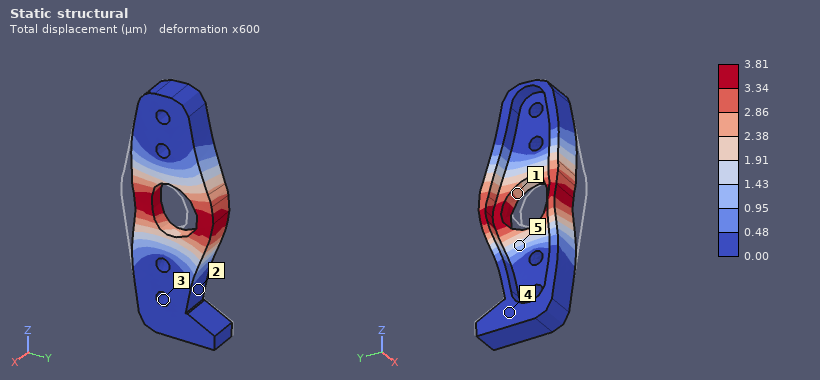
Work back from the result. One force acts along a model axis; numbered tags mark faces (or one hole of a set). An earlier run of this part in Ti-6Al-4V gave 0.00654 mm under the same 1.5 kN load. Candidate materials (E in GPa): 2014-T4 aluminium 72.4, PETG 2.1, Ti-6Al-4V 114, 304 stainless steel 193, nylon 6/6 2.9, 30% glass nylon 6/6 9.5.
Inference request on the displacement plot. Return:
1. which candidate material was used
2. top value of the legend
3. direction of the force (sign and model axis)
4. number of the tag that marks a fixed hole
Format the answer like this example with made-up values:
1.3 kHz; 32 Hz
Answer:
304 stainless steel; 3.81 µm; +Y; 3
